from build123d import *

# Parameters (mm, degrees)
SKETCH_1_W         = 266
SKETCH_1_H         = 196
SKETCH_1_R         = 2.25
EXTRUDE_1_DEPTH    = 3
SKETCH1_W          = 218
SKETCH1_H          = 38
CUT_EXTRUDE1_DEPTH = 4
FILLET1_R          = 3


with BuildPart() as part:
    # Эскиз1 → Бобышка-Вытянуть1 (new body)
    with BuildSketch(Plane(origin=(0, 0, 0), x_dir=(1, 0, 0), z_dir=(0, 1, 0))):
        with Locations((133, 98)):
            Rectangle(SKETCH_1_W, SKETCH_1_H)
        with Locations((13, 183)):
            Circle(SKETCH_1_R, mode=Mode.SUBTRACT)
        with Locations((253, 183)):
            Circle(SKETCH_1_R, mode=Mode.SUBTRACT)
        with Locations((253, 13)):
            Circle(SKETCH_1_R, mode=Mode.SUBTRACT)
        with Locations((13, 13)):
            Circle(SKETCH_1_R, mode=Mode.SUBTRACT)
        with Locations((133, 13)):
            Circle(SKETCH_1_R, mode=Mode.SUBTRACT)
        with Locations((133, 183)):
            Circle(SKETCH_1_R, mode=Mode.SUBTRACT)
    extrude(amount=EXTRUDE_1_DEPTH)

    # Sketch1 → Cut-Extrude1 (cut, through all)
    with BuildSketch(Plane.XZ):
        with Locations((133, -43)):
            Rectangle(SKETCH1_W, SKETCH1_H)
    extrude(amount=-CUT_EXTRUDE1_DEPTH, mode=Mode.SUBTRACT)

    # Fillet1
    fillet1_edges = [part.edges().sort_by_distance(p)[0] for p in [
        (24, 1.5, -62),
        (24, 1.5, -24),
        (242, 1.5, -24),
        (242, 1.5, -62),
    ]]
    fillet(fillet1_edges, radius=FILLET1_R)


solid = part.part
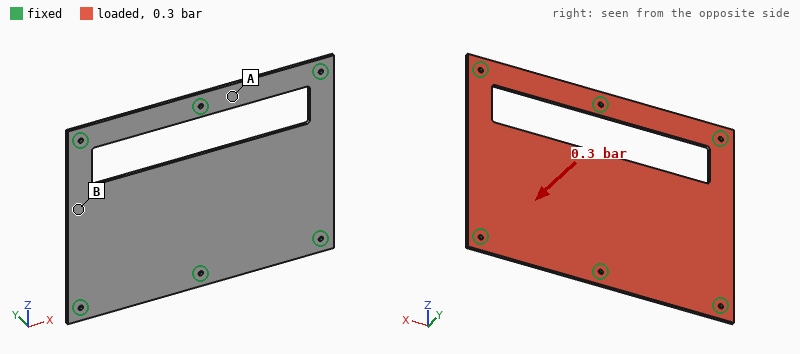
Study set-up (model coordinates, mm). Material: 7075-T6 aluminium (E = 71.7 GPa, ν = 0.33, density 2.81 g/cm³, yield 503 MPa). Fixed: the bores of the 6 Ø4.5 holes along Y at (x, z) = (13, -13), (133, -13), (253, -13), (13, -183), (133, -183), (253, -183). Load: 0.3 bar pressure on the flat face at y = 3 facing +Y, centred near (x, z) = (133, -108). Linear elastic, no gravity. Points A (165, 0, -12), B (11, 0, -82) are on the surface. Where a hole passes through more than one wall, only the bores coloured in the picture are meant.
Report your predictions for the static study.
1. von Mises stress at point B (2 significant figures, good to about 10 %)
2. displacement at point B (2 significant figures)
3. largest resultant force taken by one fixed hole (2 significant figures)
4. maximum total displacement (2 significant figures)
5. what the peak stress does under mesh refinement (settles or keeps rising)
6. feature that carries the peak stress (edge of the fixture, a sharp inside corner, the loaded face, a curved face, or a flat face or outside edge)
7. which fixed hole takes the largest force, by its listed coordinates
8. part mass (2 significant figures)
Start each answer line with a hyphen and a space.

- 45 MPa
- 0.75 mm
- 440 N
- 2.6 mm
- keeps rising
- edge of the fixture
- (133, -183)
- 370 g
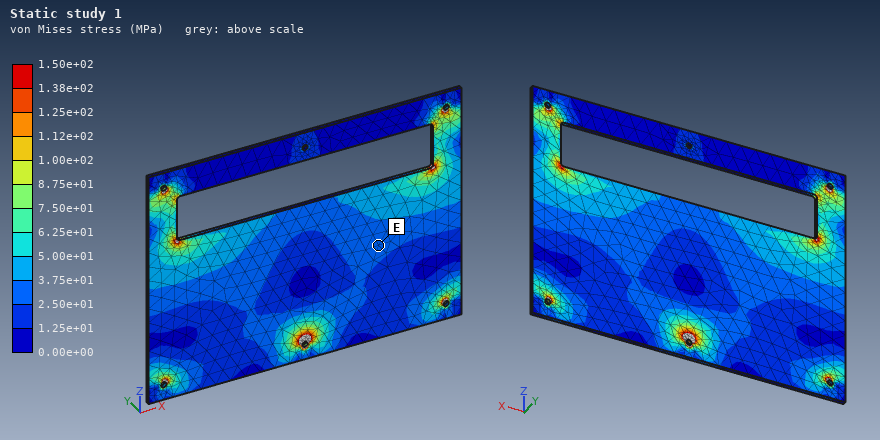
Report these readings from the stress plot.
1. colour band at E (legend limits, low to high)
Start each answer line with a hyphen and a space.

- 2.50e+01 to 3.75e+01 MPa
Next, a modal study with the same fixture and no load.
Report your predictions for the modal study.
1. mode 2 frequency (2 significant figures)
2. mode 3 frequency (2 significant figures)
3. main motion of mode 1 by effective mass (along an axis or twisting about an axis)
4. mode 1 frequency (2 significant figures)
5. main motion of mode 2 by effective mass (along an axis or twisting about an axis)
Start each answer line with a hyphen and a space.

- 440 Hz
- 610 Hz
- along Y
- 250 Hz
- twisting about Z
